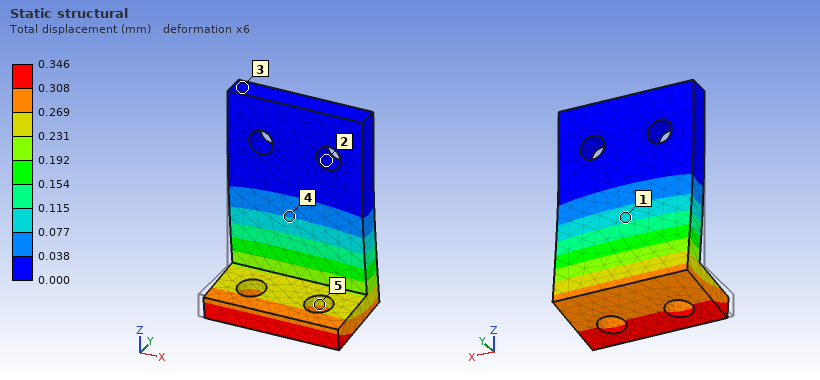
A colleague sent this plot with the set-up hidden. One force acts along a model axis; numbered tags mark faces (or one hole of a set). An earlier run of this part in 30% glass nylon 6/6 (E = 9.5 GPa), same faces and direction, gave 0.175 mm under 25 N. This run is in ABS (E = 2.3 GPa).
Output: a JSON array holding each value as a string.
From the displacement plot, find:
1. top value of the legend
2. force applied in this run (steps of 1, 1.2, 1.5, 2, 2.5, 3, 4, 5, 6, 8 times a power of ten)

["0.346 mm", "12 N"]
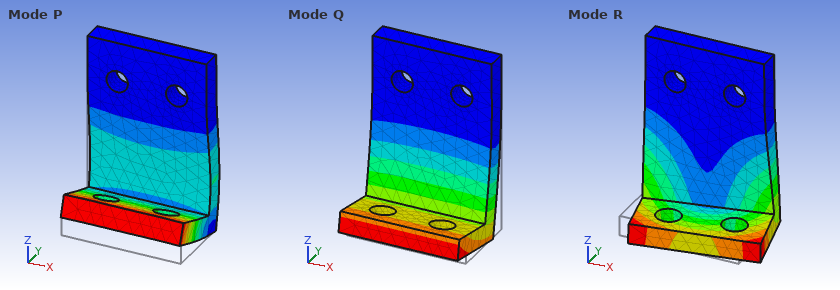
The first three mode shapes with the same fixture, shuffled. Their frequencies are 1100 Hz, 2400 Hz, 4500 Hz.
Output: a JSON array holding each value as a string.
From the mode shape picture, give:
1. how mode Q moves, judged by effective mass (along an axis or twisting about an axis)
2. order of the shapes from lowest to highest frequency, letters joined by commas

["along Y", "Q, R, P"]
